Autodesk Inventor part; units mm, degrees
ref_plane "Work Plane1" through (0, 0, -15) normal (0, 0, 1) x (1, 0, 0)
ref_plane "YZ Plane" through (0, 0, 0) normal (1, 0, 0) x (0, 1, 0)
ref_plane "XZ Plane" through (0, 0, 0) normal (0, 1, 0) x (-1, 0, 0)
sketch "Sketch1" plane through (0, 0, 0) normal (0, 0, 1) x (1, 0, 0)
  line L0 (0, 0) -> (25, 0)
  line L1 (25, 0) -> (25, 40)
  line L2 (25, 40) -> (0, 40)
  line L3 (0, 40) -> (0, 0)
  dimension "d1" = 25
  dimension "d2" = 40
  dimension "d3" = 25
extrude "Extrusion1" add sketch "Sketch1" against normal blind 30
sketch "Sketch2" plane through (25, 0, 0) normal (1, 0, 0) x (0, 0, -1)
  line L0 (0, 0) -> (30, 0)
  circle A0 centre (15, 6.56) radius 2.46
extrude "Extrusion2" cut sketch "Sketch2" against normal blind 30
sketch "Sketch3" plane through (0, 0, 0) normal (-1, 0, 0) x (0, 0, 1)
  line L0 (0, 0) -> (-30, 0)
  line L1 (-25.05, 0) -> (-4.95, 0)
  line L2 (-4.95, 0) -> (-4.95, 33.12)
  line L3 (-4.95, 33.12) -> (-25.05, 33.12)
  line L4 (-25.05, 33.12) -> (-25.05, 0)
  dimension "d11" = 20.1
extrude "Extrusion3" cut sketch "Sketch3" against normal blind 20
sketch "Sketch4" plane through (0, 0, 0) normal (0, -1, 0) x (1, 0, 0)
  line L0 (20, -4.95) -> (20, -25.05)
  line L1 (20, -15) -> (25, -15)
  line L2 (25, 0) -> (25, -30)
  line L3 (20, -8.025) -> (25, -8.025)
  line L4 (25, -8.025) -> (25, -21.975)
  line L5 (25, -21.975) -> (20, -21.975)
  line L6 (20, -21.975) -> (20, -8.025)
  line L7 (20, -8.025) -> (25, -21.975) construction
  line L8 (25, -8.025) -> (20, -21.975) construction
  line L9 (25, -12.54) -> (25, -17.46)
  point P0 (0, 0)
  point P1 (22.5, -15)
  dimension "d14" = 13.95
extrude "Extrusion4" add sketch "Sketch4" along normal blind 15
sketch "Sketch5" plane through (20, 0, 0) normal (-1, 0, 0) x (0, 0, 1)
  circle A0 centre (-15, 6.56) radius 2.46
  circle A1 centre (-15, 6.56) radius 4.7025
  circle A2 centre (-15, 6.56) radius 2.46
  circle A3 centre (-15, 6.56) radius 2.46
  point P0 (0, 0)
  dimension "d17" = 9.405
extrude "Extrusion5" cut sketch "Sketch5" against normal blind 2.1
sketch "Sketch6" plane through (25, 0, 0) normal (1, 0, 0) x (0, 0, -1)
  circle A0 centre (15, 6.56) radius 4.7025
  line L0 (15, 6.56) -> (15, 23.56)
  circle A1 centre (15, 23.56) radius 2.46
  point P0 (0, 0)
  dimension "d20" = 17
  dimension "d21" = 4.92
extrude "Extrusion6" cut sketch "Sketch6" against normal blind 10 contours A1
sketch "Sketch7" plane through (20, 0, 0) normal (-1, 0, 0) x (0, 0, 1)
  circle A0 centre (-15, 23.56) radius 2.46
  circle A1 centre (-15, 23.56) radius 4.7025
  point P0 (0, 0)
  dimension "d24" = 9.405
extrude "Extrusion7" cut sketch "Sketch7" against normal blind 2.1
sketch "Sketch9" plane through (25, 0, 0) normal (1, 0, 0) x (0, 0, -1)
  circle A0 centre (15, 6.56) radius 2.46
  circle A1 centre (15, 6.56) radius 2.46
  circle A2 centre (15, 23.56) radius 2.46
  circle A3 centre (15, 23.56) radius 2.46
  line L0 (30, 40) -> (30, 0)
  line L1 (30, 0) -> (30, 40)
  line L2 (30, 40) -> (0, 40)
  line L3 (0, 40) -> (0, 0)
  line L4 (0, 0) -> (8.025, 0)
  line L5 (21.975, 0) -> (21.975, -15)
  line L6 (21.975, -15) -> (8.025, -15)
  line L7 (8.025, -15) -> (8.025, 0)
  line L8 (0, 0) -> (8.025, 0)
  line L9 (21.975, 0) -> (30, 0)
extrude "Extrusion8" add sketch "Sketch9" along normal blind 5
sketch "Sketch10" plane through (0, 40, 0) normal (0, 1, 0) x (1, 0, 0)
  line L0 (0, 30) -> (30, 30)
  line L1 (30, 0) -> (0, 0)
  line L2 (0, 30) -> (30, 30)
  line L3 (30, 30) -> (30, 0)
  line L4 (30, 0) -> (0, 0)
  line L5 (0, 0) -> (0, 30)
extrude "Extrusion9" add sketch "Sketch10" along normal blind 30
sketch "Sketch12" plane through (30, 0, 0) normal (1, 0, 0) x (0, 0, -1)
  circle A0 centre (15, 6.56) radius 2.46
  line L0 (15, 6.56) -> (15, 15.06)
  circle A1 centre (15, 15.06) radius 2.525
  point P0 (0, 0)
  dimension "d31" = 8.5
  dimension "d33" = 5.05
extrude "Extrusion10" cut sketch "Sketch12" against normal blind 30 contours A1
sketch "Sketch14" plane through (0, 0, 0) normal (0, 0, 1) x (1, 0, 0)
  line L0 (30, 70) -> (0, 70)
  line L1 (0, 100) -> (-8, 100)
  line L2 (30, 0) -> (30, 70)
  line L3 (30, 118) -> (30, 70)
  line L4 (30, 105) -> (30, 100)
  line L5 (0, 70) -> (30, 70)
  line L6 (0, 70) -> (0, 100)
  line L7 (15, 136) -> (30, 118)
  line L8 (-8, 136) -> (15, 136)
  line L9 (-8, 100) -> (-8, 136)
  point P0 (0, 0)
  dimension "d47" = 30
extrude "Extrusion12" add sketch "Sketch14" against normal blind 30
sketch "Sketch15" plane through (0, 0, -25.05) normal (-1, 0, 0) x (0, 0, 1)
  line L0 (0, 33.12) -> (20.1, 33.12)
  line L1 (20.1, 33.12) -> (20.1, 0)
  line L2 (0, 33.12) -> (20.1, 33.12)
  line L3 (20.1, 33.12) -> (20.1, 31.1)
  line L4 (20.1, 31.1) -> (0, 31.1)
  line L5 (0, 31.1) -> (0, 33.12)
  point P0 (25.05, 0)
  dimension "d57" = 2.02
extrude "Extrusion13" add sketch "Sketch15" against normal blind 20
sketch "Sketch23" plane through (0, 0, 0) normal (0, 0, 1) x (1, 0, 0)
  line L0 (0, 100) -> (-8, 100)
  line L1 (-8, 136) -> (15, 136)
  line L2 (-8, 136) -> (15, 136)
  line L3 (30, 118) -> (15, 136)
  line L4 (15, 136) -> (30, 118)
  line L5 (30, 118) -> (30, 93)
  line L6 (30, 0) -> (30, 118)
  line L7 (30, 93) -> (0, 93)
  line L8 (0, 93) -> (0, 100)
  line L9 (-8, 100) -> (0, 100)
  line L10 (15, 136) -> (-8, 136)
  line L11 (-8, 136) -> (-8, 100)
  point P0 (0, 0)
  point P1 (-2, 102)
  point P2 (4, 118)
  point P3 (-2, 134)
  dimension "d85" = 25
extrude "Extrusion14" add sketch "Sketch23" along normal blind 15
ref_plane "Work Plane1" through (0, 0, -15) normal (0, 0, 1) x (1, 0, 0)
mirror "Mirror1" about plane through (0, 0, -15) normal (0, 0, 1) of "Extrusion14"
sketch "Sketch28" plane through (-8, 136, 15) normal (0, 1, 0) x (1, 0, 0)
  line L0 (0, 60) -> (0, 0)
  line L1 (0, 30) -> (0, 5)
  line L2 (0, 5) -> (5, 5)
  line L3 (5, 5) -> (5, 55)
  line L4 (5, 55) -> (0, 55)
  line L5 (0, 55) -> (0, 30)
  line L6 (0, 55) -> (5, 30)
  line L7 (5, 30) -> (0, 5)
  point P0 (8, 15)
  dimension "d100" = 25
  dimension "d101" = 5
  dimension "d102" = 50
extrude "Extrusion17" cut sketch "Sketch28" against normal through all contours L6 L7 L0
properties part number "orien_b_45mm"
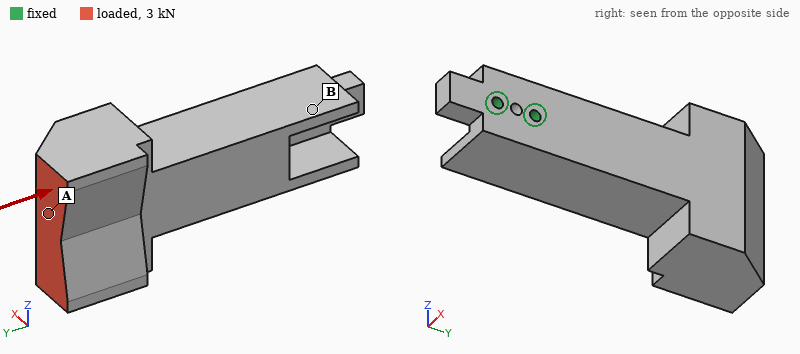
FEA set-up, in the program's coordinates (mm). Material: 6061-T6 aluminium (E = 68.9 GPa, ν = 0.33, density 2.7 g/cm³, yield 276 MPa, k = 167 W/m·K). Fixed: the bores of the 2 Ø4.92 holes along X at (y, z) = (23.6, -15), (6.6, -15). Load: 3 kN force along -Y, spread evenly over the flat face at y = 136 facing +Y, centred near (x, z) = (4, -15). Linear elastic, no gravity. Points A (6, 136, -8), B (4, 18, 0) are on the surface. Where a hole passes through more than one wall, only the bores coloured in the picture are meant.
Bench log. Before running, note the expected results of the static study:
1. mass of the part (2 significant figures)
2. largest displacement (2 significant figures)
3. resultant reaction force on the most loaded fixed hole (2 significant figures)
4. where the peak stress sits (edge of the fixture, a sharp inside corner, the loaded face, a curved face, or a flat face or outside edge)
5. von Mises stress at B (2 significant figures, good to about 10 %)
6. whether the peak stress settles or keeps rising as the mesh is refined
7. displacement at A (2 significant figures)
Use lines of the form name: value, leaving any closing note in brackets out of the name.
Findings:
mass of the part: 420 g
largest displacement: 0.20 mm
resultant reaction force on the most loaded fixed hole: 3.0 kN
where the peak stress sits: edge of the fixture
von Mises stress at B: 14 MPa
whether the peak stress settles or keeps rising as the mesh is refined: keeps rising
displacement at A: 0.19 mm
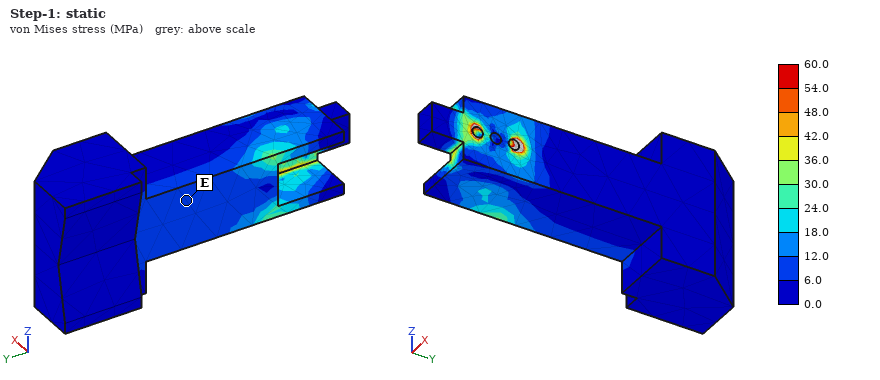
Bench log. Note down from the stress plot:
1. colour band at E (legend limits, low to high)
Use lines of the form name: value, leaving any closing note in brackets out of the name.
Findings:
colour band at E: 6.0 to 12.0 MPa
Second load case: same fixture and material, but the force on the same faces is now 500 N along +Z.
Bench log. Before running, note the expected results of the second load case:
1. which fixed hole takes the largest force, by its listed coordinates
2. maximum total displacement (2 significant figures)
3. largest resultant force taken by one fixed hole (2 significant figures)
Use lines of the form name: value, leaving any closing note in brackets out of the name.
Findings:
which fixed hole takes the largest force, by its listed coordinates: (23.6, -15)
maximum total displacement: 0.15 mm
largest resultant force taken by one fixed hole: 2.9 kN
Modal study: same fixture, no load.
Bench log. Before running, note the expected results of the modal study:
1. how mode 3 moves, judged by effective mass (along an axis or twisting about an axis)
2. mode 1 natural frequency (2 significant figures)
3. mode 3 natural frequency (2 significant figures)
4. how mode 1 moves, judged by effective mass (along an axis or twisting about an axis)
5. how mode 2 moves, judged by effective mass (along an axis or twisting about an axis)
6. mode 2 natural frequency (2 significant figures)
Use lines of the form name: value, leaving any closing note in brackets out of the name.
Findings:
how mode 3 moves, judged by effective mass: twisting about Y
mode 1 natural frequency: 650 Hz
mode 3 natural frequency: 1800 Hz
how mode 1 moves, judged by effective mass: along X
how mode 2 moves, judged by effective mass: along Z
mode 2 natural frequency: 750 Hz
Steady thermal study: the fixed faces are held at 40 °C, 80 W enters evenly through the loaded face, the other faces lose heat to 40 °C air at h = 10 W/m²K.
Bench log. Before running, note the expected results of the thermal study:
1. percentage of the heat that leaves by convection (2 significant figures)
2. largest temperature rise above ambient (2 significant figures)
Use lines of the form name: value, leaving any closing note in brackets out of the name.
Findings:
percentage of the heat that leaves by convection: 10 %
largest temperature rise above ambient: 61 K
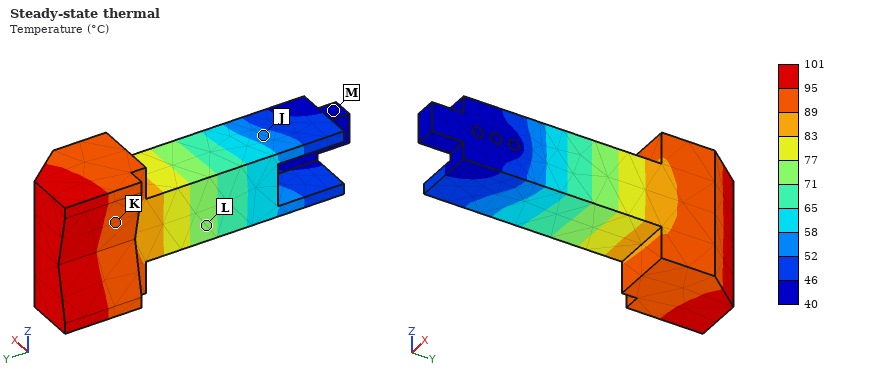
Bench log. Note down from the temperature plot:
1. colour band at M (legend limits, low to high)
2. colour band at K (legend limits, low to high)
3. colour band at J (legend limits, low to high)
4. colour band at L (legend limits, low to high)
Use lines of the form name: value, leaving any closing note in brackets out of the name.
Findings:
colour band at M: 40 to 46 °C
colour band at K: 89 to 95 °C
colour band at J: 52 to 58 °C
colour band at L: 71 to 77 °C
